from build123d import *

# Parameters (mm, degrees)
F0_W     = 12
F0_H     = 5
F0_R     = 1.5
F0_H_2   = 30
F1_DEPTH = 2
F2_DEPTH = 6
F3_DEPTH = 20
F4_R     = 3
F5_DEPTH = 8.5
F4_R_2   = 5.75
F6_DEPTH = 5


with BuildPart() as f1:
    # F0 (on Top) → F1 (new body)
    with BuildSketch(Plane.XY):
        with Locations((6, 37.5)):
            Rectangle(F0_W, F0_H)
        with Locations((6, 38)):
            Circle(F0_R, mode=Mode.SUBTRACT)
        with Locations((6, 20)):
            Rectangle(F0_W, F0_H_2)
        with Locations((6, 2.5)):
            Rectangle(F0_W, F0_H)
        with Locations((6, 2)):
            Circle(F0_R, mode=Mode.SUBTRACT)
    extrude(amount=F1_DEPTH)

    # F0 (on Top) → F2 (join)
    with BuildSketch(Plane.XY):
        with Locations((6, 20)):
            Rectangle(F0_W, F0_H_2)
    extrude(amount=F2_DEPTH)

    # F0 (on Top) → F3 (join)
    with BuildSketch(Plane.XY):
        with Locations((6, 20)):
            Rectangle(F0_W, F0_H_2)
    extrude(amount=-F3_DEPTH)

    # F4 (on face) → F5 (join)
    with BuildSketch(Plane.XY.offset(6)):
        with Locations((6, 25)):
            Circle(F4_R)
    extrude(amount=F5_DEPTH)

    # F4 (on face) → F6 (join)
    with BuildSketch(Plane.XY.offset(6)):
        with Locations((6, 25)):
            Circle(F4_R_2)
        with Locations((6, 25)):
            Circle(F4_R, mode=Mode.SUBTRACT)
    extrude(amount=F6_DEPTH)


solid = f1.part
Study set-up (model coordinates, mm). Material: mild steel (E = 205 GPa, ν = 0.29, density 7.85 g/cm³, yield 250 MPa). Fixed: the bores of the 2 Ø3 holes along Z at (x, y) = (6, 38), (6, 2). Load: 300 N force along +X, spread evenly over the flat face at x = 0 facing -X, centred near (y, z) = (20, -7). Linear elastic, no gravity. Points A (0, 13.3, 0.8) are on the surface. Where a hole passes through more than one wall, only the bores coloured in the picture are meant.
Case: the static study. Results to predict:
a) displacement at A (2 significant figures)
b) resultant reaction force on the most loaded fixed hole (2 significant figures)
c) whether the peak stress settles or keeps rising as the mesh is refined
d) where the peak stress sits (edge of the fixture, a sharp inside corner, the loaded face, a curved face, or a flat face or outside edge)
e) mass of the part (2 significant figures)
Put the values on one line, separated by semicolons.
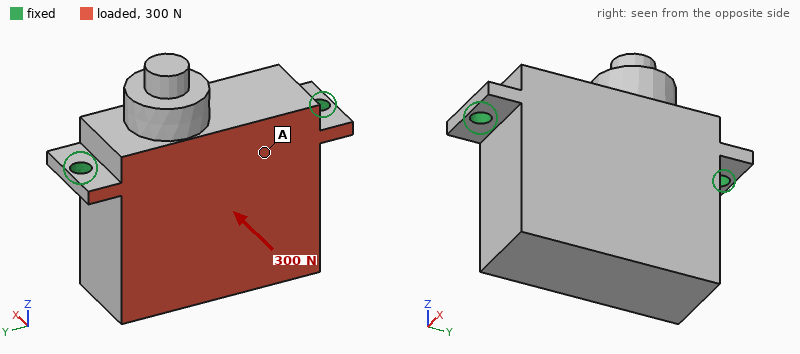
5.9 µm; 150 N; keeps rising; edge of the fixture; 80 g
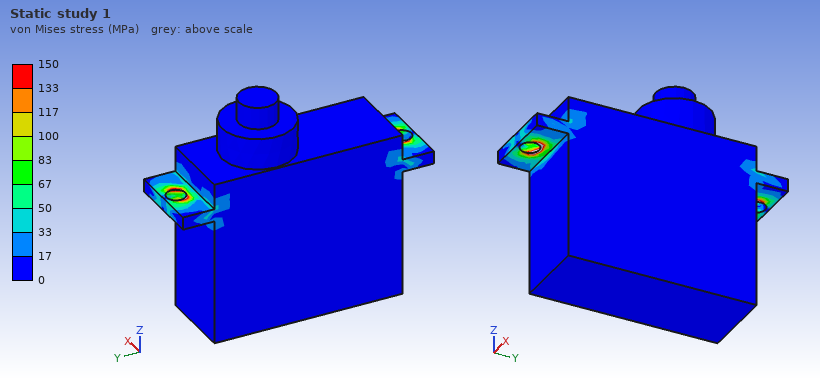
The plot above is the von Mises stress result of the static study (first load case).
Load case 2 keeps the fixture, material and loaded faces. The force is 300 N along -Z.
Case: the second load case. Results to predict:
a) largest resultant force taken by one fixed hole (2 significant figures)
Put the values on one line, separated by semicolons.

150 N
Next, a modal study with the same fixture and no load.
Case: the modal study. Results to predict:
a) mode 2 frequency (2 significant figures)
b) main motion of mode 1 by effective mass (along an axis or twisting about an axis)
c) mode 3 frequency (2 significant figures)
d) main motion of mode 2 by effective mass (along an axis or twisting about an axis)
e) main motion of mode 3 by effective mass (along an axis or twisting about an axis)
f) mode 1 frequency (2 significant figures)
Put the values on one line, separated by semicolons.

11 kHz; along X; 12 kHz; along Z; along Y; 2400 Hz
